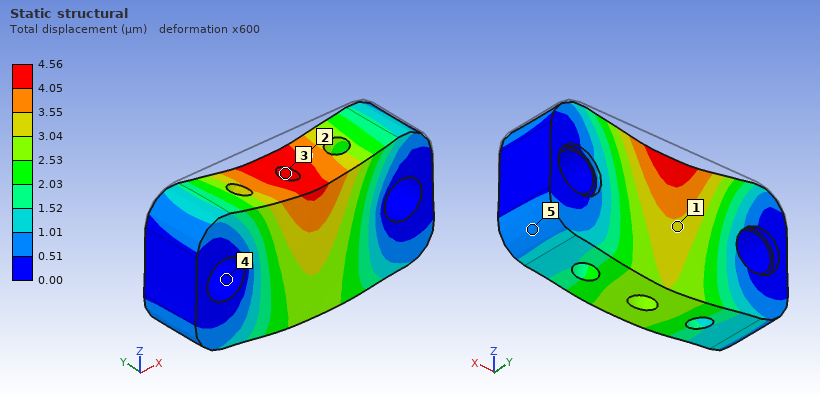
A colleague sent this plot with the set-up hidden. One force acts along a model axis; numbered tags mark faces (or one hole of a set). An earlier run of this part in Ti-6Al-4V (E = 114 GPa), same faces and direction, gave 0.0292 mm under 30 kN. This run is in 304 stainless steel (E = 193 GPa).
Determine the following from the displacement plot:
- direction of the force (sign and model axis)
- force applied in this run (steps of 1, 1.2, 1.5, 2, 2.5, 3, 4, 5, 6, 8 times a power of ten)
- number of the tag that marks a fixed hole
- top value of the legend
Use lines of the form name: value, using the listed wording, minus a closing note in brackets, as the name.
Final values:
direction of the force: -Z
force applied in this run: 8 kN
number of the tag that marks a fixed hole: 4
top value of the legend: 4.56 µm
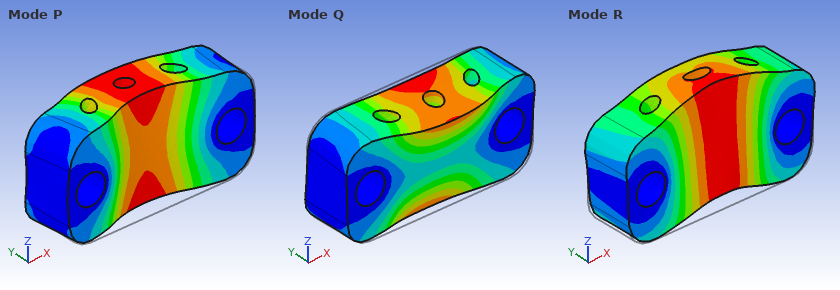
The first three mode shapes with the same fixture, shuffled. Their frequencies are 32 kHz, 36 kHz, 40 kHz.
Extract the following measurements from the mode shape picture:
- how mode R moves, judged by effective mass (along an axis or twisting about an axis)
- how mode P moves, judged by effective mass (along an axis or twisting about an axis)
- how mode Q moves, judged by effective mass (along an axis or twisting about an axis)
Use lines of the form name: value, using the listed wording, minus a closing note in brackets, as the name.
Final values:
how mode R moves, judged by effective mass: along Z
how mode P moves, judged by effective mass: along Y
how mode Q moves, judged by effective mass: twisting about X
